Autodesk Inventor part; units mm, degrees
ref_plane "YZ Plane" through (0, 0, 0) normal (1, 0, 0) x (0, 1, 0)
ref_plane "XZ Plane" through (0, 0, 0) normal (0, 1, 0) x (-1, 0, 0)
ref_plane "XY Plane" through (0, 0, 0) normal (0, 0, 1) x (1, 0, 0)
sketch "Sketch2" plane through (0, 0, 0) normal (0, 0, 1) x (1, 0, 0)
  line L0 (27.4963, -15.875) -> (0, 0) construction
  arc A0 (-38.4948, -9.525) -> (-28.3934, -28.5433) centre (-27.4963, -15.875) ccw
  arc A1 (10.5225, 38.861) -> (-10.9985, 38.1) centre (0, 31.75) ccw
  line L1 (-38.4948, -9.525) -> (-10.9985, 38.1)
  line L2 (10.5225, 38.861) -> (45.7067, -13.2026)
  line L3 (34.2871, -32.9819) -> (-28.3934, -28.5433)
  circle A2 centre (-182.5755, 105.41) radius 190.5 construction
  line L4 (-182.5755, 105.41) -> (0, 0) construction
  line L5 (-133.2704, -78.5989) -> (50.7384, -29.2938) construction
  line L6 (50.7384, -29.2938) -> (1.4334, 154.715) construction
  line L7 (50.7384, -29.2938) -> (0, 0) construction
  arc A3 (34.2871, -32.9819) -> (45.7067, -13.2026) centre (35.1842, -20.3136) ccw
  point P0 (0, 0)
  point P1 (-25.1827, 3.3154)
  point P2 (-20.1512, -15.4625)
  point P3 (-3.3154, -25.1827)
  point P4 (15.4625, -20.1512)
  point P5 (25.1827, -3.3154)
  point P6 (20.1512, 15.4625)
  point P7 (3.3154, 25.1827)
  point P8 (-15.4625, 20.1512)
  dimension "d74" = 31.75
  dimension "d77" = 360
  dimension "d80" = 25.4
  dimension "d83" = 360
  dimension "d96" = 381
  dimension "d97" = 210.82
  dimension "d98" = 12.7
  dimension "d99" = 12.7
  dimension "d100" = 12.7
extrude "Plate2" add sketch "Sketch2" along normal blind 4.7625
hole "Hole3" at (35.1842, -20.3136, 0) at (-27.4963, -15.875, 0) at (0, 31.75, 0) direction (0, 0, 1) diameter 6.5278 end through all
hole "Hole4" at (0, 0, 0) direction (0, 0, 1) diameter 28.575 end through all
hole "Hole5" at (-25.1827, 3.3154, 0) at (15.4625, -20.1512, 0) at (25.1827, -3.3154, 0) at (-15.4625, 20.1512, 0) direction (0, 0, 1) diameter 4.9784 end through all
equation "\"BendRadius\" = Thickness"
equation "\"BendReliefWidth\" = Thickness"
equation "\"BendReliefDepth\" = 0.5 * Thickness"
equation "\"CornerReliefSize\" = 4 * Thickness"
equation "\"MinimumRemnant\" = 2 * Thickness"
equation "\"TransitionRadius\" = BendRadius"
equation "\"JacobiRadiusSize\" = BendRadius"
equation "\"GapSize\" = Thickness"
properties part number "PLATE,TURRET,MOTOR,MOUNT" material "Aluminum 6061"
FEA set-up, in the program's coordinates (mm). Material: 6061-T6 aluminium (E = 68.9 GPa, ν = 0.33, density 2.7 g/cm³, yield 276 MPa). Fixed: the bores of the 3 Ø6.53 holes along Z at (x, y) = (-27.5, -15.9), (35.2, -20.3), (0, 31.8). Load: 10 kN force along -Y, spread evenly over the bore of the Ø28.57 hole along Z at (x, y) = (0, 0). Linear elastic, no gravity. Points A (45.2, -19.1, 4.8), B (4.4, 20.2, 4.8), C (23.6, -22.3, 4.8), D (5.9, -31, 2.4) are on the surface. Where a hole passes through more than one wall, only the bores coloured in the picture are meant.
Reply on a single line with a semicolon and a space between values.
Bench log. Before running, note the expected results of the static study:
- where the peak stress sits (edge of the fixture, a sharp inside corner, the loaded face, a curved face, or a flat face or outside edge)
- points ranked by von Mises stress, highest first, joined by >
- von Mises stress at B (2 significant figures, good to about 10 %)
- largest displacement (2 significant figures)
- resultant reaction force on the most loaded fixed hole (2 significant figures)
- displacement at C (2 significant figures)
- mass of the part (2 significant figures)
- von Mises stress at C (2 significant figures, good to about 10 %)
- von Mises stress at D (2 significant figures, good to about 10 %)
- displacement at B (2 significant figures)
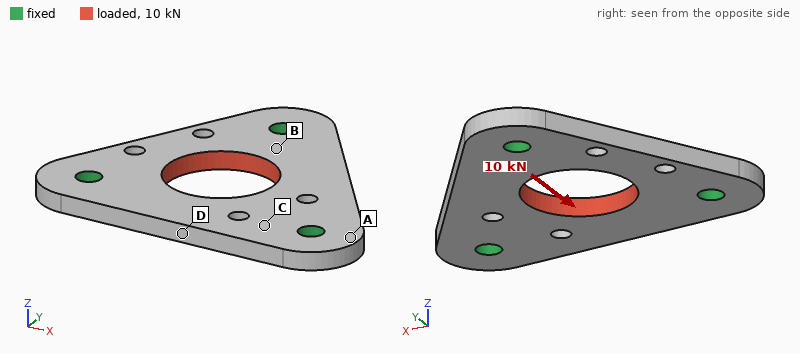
edge of the fixture; D > B > C > A; 46 MPa; 40 µm; 3.8 kN; 15 µm; 45 g; 33 MPa; 62 MPa; 7.8 µm
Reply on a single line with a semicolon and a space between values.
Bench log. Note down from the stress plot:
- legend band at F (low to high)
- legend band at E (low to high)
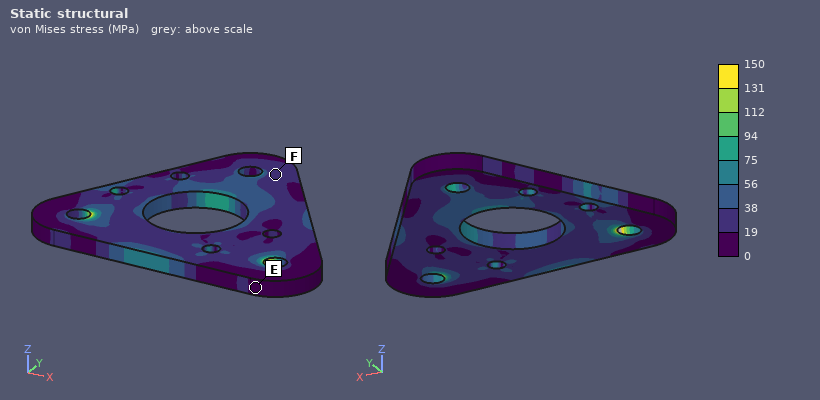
19 to 38 MPa; 0 to 19 MPa
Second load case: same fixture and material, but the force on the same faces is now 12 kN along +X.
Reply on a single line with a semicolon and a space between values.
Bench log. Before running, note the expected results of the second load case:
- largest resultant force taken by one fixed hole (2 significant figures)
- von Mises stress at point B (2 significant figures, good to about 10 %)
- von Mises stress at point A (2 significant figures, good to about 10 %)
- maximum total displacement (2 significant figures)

4.4 kN; 34 MPa; 17 MPa; 39 µm
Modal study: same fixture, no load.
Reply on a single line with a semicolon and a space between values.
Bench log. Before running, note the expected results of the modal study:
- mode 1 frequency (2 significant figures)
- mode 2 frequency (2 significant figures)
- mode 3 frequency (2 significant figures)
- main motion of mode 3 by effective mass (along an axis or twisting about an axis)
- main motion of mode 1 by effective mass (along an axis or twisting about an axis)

6700 Hz; 7100 Hz; 9000 Hz; along Z; along Z
